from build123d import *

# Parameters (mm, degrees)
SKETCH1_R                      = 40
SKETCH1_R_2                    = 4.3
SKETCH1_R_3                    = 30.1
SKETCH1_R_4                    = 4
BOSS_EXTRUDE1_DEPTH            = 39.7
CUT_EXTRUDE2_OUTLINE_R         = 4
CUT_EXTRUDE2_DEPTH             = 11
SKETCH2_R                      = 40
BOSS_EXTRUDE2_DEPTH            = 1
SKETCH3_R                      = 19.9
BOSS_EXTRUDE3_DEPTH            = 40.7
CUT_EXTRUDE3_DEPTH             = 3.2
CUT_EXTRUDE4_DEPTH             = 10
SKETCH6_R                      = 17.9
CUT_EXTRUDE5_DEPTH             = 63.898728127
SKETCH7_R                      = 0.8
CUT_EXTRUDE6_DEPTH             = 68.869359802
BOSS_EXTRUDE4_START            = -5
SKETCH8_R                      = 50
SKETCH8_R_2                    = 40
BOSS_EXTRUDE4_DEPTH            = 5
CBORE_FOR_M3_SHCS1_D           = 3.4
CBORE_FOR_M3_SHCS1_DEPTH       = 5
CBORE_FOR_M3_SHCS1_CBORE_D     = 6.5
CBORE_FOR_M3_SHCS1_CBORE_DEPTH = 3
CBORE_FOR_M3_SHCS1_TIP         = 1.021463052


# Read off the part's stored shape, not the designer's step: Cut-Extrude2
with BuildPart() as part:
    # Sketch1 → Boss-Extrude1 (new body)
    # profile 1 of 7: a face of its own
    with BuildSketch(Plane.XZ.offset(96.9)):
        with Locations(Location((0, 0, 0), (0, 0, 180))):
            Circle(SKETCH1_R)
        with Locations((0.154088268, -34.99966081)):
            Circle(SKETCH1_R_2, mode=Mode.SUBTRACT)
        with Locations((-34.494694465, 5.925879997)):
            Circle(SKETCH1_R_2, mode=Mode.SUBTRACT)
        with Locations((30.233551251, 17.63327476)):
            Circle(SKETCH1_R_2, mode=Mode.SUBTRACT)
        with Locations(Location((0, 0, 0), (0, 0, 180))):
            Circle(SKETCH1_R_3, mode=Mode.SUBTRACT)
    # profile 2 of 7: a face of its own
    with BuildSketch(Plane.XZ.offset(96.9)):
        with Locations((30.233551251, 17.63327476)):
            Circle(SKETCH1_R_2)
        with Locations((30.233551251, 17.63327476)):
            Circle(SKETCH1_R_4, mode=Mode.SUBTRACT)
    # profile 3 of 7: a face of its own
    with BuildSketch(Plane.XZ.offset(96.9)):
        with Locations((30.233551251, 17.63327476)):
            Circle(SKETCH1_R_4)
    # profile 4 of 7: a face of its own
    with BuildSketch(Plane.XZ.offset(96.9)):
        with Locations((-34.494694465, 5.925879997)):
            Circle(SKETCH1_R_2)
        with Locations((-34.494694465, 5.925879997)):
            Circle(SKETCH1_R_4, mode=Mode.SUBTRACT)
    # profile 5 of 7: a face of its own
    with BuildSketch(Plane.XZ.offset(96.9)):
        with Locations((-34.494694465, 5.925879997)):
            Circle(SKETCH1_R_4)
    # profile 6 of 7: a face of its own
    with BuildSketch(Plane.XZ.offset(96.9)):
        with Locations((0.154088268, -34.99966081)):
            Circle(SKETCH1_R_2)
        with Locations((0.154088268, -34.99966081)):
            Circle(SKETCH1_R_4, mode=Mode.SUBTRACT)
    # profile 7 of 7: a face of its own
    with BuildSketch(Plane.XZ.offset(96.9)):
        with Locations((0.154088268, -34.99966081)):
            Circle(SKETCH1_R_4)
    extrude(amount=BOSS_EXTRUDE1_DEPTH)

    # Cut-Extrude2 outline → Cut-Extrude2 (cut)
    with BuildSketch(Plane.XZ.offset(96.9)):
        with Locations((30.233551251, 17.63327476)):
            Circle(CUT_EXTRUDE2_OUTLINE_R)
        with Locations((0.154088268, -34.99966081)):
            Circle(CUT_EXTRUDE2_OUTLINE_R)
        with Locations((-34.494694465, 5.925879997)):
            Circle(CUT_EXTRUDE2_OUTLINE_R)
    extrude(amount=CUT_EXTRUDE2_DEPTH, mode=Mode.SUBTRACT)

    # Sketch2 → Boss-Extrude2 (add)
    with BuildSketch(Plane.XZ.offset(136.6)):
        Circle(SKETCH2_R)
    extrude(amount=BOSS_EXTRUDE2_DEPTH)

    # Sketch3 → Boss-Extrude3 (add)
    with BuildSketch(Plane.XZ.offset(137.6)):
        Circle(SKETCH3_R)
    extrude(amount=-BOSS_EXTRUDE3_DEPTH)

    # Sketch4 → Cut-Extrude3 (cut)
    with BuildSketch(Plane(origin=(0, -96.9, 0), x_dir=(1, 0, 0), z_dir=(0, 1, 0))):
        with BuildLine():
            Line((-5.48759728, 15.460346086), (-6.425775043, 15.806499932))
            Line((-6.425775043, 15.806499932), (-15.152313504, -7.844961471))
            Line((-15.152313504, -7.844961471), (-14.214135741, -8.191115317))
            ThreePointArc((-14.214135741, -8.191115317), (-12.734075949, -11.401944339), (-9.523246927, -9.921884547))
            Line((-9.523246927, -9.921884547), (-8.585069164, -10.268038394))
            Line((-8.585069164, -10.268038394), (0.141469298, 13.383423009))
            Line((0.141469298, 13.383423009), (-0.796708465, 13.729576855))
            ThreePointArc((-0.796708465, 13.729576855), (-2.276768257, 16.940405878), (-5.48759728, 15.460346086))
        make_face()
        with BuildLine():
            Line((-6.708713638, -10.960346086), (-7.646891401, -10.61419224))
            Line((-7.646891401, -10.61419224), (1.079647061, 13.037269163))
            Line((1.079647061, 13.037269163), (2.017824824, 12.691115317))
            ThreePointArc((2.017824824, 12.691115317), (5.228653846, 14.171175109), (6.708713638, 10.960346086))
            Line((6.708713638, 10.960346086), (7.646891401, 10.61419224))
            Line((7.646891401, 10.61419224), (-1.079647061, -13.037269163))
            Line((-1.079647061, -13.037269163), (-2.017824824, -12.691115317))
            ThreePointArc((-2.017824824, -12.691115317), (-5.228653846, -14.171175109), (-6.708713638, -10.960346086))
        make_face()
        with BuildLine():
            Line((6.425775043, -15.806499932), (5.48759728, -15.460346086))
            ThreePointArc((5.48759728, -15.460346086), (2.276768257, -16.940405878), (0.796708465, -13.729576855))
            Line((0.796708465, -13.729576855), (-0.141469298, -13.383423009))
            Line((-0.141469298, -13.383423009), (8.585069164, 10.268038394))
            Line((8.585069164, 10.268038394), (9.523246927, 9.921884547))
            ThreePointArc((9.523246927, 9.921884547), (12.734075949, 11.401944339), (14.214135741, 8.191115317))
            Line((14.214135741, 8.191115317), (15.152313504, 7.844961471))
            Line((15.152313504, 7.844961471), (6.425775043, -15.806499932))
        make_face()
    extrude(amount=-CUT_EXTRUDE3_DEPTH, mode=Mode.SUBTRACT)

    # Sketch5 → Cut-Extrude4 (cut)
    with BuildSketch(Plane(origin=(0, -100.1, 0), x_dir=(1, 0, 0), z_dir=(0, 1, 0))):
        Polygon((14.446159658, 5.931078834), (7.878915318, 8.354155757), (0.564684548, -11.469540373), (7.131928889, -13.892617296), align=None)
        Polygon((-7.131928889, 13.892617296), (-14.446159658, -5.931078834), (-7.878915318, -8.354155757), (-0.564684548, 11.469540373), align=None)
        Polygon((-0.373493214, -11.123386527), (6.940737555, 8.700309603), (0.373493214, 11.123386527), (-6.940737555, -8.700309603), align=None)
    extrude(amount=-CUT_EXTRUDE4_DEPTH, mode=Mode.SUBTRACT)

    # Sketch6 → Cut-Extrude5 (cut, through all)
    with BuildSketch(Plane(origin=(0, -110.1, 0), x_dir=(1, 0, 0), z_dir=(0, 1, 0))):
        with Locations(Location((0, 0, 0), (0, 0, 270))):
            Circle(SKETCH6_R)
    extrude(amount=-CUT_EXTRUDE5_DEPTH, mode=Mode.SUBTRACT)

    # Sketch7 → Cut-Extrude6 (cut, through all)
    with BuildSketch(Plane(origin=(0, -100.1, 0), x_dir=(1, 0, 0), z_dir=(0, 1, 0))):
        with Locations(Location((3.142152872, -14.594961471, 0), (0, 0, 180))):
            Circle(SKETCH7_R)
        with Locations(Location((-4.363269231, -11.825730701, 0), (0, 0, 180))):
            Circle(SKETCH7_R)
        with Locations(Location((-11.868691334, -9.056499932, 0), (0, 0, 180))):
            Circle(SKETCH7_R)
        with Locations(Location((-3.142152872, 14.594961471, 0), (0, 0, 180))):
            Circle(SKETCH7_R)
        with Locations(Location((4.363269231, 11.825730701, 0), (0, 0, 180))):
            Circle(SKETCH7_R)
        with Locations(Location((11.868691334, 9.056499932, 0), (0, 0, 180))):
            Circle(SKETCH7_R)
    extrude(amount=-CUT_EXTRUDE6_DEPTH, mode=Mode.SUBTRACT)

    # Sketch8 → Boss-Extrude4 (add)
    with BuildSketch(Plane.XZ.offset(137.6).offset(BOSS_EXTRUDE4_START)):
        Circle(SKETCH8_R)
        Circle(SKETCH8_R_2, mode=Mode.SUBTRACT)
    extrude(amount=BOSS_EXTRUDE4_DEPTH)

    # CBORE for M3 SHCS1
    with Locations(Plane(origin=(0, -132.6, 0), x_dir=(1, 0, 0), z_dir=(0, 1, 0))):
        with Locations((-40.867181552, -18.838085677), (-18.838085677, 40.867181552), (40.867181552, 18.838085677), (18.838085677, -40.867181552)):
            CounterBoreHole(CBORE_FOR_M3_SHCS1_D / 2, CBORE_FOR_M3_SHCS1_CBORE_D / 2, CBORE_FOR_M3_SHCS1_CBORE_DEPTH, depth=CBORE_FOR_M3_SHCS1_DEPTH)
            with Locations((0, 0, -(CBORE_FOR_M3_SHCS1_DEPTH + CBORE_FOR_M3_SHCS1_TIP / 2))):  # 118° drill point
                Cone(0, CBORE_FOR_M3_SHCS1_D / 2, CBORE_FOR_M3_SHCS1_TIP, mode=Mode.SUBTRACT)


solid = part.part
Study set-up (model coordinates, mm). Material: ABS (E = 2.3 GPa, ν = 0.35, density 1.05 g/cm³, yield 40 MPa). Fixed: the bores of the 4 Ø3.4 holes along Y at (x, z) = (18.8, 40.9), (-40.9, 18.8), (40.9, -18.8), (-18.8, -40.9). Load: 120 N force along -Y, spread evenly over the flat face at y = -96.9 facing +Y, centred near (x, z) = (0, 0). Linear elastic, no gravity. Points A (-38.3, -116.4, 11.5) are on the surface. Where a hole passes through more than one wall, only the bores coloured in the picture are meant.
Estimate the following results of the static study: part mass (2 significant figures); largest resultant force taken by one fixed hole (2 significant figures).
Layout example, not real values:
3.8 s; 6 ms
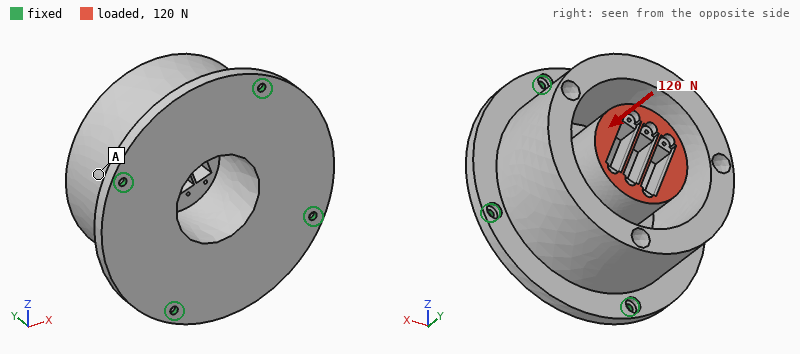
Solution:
120 g; 42 N
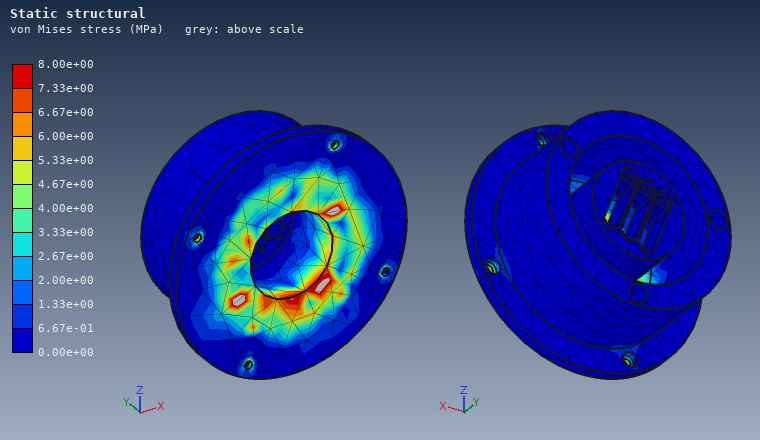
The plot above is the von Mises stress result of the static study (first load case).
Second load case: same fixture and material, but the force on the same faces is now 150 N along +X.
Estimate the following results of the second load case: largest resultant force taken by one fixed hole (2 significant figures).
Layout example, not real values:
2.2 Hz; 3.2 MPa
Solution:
97 N
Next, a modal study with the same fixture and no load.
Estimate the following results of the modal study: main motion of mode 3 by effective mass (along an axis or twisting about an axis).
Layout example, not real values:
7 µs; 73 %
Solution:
along Y
